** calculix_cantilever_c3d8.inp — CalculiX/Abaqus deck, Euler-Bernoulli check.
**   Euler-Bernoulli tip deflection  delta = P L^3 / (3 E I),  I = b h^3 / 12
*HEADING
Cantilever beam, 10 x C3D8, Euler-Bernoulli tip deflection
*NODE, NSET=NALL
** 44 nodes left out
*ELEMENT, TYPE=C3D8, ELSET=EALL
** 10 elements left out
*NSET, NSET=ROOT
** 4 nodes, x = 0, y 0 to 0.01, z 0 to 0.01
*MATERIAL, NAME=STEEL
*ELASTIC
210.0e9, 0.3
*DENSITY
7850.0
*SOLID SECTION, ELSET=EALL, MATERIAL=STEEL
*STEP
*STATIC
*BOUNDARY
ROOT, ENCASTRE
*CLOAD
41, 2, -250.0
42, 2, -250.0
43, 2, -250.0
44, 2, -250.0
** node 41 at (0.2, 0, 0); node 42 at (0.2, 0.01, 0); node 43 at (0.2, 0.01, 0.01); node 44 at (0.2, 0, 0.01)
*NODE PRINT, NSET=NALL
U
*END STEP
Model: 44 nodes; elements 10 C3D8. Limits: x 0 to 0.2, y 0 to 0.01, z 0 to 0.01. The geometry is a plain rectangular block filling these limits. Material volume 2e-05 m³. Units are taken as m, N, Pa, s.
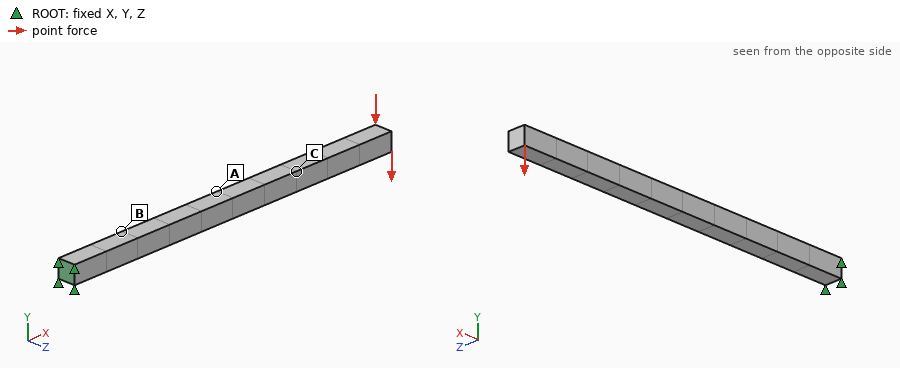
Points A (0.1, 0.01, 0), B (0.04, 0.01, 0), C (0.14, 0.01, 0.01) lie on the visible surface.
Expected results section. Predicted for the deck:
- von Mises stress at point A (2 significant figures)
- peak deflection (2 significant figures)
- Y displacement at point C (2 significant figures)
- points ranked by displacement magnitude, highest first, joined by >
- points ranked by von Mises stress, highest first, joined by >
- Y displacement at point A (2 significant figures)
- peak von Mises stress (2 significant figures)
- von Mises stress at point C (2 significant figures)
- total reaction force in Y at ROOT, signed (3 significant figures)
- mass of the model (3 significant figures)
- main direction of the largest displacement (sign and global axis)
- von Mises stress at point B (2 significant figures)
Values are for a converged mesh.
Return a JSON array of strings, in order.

["6.0e+08 Pa", "0.015 m", "-0.0084 m", "C > A > B", "B > A > C", "-0.0046 m", "1.1e+09 Pa", "3.6e+08 Pa", "1000 N", "0.157 kg", "-Y", "9.5e+08 Pa"]
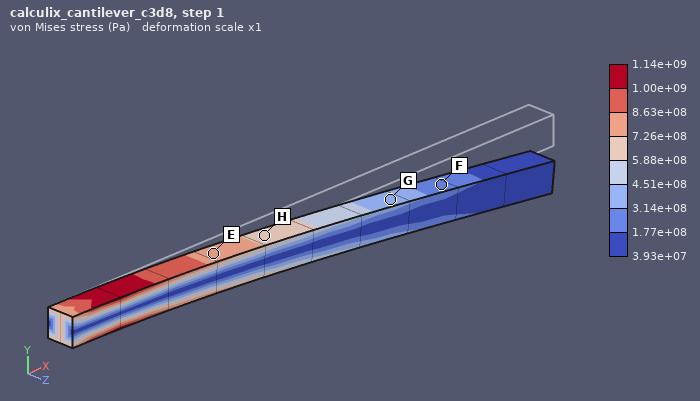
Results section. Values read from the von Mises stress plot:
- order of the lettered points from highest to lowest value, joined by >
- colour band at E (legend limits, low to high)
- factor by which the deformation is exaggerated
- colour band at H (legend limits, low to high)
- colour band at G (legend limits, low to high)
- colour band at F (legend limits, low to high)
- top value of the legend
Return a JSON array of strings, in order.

["E > H > G > F", "7.26e+08 to 8.63e+08 Pa", "1", "5.88e+08 to 7.26e+08 Pa", "3.14e+08 to 4.51e+08 Pa", "1.77e+08 to 3.14e+08 Pa", "1.14e+09 Pa"]
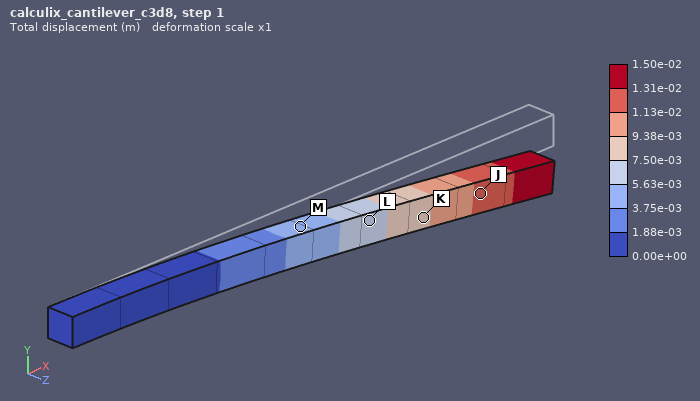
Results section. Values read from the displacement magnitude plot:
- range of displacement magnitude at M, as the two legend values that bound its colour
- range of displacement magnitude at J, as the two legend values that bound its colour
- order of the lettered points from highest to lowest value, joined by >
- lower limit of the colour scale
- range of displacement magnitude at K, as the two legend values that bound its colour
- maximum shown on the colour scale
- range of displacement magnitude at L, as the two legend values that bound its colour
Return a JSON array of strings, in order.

["3.75e-03 to 5.63e-03 m", "1.13e-02 to 1.31e-02 m", "J > K > L > M", "0.00e+00 m", "7.50e-03 to 9.38e-03 m", "1.50e-02 m", "5.63e-03 to 7.50e-03 m"]
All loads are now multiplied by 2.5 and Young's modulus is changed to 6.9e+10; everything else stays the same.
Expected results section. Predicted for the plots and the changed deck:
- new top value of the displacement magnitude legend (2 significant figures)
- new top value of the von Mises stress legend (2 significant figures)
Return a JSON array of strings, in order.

["0.11 m", "2.8e+09 Pa"]
